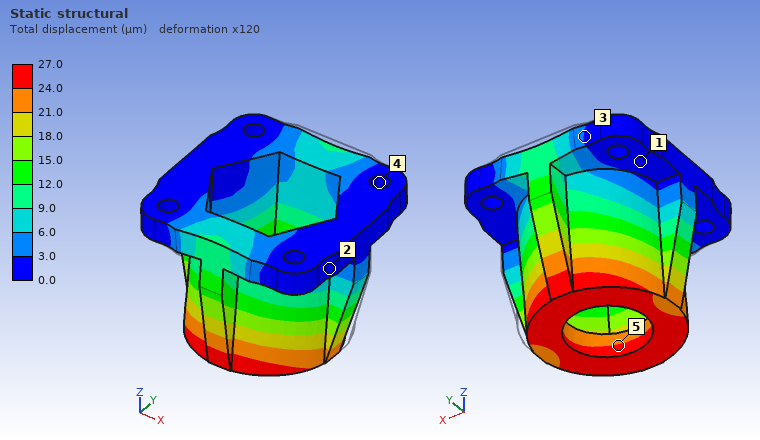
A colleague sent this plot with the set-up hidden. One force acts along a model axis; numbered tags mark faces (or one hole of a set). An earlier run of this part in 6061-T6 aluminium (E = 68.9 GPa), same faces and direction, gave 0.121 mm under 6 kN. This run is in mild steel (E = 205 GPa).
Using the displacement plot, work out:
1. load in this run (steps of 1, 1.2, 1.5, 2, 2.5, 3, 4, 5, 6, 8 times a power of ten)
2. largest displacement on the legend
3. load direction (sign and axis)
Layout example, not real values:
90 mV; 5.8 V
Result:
4 kN; 27.0 µm; -Y
